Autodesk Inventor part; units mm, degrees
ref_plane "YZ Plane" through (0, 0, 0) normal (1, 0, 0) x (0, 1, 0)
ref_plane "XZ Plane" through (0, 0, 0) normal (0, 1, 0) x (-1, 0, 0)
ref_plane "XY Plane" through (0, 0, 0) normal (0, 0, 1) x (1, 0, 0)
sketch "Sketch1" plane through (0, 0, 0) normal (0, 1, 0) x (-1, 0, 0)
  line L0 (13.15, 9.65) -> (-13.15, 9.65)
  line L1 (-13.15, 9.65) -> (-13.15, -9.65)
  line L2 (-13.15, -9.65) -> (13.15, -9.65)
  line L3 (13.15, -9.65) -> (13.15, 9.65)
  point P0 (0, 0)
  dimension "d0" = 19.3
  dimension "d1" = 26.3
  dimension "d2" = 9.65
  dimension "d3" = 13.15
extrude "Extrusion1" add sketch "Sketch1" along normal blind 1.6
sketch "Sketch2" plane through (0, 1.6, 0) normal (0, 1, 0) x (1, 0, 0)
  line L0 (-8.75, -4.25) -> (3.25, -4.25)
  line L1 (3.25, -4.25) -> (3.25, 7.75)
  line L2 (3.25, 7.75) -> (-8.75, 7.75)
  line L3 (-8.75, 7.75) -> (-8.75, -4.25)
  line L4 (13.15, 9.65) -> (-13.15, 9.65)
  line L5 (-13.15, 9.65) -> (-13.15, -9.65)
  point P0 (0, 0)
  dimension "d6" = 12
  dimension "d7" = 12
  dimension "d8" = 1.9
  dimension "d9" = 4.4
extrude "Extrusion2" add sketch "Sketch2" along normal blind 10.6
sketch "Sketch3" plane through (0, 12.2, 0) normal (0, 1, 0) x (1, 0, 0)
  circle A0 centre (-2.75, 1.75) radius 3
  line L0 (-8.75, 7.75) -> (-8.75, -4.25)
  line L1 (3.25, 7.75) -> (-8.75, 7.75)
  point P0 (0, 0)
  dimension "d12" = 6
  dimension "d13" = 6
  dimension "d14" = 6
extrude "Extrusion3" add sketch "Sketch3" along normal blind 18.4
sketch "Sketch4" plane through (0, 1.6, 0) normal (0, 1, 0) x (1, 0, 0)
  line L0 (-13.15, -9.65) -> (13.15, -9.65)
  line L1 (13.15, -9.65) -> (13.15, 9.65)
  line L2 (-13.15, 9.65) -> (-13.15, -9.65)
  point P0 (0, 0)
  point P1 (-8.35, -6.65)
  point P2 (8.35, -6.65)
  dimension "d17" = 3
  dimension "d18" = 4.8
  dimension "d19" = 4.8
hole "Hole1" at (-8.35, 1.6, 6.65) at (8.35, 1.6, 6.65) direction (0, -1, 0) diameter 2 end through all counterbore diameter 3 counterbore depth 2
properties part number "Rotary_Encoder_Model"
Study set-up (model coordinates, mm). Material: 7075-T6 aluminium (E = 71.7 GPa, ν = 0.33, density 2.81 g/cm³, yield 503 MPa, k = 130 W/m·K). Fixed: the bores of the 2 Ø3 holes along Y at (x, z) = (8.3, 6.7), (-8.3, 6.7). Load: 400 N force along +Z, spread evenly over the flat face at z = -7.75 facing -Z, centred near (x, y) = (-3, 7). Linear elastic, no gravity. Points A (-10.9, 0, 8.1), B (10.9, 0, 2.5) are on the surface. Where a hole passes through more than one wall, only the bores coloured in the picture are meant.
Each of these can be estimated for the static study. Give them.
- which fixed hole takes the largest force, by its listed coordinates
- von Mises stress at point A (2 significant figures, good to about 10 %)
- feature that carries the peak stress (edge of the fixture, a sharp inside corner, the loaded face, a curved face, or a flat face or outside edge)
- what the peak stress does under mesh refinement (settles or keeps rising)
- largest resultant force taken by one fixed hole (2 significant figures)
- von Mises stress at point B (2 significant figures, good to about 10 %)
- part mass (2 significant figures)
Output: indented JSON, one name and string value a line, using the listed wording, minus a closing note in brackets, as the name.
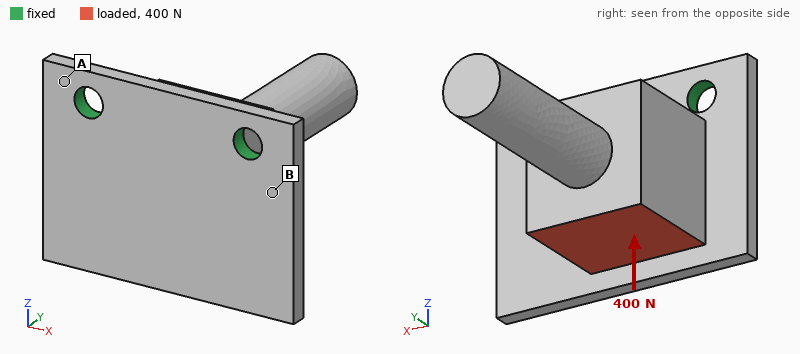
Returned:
{
  "which fixed hole takes the largest force, by its listed coordinates": "(-8.3, 6.7)",
  "von Mises stress at point A": "34 MPa",
  "feature that carries the peak stress": "edge of the fixture",
  "what the peak stress does under mesh refinement": "keeps rising",
  "largest resultant force taken by one fixed hole": "280 N",
  "von Mises stress at point B": "110 MPa",
  "part mass": "8.0 g"
}
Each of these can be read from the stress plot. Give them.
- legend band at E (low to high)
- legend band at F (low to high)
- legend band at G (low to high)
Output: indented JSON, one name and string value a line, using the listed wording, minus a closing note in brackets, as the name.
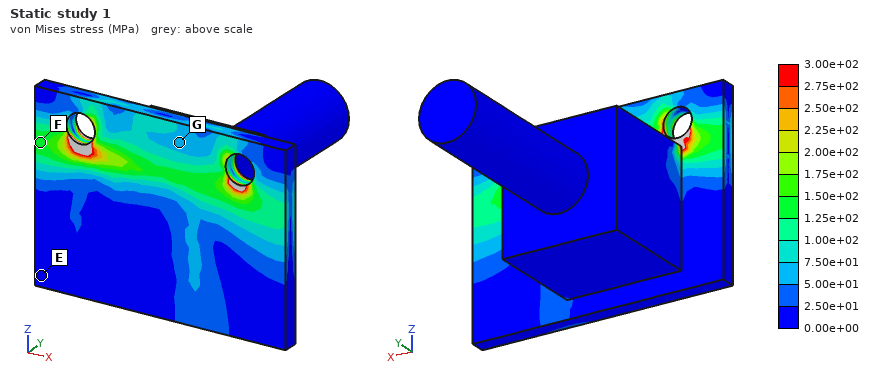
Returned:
{
  "legend band at E": "0.00e+00 to 2.50e+01 MPa",
  "legend band at F": "1.25e+02 to 1.50e+02 MPa",
  "legend band at G": "5.00e+01 to 7.50e+01 MPa"
}
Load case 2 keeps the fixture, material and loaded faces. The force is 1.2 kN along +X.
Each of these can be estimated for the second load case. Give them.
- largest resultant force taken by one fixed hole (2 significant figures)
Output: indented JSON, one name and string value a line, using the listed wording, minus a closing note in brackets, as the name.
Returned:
{
  "largest resultant force taken by one fixed hole": "1.2 kN"
}
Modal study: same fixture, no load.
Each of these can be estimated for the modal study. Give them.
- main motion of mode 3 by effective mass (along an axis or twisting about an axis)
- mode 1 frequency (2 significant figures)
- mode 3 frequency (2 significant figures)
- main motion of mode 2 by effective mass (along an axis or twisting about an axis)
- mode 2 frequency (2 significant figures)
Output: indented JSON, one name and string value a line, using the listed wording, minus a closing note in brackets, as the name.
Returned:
{
  "main motion of mode 3 by effective mass": "along Y",
  "mode 1 frequency": "1800 Hz",
  "mode 3 frequency": "12 kHz",
  "main motion of mode 2 by effective mass": "along X",
  "mode 2 frequency": "5200 Hz"
}
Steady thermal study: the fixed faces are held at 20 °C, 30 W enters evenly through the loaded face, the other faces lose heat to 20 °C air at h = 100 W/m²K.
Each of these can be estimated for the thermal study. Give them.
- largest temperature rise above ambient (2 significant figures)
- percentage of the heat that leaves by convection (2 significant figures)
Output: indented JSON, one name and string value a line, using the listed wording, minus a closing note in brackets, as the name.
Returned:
{
  "largest temperature rise above ambient": "49 K",
  "percentage of the heat that leaves by convection": "18 %"
}
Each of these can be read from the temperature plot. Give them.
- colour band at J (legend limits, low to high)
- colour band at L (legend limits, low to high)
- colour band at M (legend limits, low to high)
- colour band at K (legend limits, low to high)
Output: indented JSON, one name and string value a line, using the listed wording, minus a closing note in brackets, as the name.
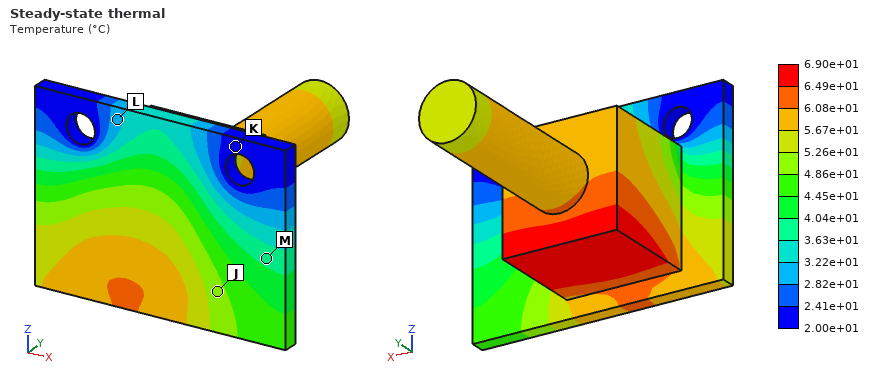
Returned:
{
  "colour band at J": "4.86e+01 to 5.26e+01 °C",
  "colour band at L": "2.82e+01 to 3.22e+01 °C",
  "colour band at M": "3.63e+01 to 4.04e+01 °C",
  "colour band at K": "2.00e+01 to 2.41e+01 °C"
}
